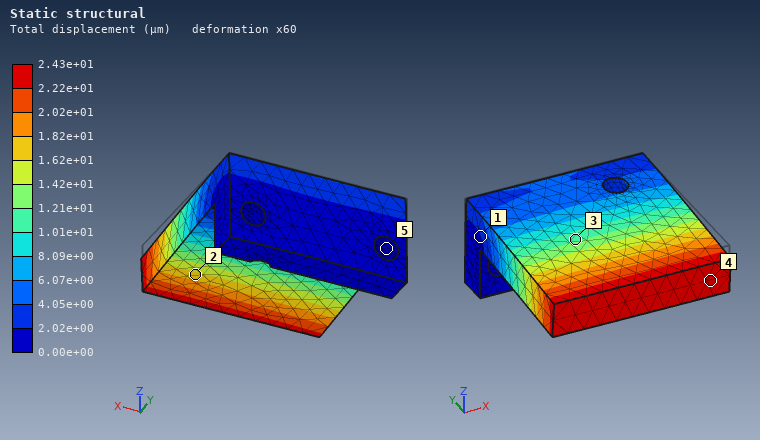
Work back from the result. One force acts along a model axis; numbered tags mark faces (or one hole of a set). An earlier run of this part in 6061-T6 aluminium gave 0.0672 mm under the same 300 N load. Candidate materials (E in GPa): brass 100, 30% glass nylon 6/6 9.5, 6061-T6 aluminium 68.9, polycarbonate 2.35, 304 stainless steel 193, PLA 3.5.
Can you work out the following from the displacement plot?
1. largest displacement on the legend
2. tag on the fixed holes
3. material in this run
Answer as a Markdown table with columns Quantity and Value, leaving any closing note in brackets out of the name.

| Quantity | Value |
|---|---|
| largest displacement on the legend | 2.43e+01 µm |
| tag on the fixed holes | 5 |
| material in this run | 304 stainless steel |
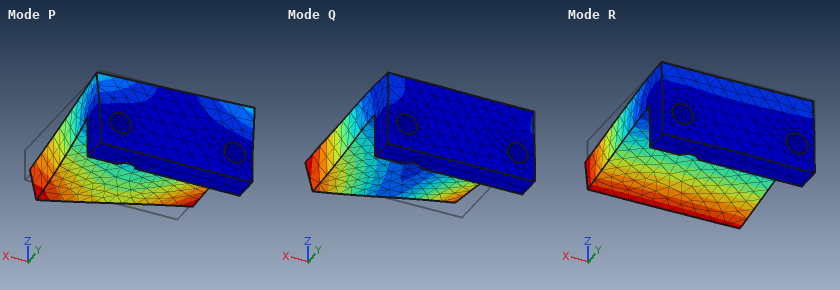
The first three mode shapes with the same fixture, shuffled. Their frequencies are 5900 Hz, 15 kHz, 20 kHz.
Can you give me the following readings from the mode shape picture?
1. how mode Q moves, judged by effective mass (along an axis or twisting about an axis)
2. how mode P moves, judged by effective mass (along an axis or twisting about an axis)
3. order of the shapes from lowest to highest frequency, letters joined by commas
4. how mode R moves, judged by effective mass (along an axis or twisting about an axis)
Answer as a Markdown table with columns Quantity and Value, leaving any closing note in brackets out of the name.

| Quantity | Value |
|---|---|
| how mode Q moves, judged by effective mass | along X |
| how mode P moves, judged by effective mass | along X |
| order of the shapes from lowest to highest frequency, letters joined by commas | R, P, Q |
| how mode R moves, judged by effective mass | along Z |
